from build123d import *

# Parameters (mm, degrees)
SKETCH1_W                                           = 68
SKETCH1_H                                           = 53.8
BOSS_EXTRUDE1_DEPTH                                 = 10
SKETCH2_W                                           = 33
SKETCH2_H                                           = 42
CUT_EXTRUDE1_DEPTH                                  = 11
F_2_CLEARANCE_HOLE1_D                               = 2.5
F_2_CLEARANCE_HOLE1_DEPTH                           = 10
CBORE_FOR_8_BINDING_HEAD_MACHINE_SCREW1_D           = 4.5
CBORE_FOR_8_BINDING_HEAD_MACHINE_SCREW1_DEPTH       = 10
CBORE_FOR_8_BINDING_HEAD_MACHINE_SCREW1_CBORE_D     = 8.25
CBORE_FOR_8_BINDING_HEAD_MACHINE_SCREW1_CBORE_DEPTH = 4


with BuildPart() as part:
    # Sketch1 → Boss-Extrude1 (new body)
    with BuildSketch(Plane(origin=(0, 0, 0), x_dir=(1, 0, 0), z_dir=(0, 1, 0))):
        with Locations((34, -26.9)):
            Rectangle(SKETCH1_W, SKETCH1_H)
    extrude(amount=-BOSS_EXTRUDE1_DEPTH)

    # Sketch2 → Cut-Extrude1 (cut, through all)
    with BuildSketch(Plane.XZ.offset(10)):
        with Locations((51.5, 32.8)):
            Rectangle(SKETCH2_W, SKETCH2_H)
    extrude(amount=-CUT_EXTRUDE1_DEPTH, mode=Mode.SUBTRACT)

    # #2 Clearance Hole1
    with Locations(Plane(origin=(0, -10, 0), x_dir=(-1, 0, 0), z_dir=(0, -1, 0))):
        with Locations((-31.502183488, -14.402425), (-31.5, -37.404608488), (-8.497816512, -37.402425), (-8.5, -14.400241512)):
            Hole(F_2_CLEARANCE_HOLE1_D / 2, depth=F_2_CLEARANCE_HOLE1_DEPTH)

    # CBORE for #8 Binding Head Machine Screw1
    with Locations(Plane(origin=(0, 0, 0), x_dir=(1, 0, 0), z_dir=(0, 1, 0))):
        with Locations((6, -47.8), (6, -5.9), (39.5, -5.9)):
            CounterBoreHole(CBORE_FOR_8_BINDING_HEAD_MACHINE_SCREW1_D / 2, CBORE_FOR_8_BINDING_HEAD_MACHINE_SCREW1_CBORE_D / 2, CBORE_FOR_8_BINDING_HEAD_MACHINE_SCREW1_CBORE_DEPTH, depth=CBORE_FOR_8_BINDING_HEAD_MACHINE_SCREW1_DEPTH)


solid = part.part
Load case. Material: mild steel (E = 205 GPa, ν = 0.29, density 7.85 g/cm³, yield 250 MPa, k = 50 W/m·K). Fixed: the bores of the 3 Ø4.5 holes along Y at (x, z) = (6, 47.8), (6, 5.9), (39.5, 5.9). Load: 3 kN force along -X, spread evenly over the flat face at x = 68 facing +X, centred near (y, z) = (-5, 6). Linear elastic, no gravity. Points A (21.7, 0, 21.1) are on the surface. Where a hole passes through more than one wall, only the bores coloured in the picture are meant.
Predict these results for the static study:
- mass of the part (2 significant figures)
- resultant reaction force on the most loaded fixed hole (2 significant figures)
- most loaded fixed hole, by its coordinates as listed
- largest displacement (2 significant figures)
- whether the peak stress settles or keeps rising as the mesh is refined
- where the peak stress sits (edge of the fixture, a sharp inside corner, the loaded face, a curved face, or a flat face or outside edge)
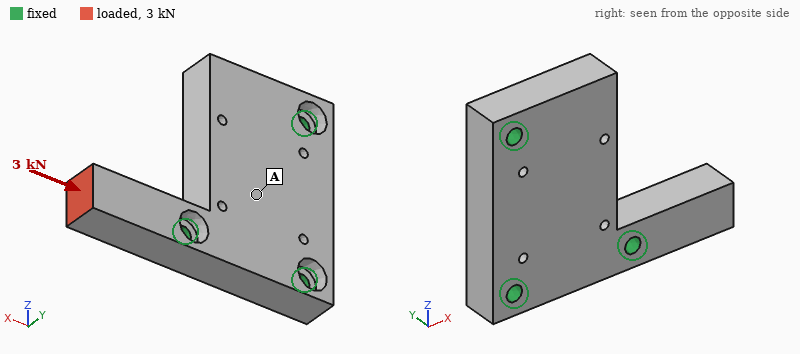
170 g
2.7 kN
(39.5, 5.9)
9.2 µm
keeps rising
edge of the fixture
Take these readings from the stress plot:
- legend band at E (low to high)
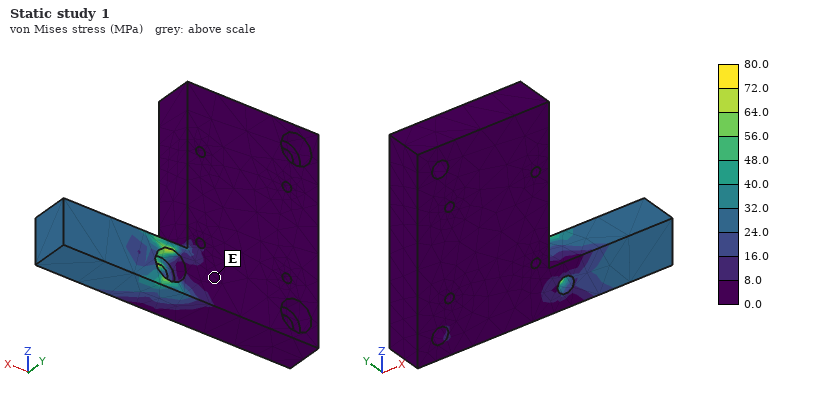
0.0 to 8.0 MPa
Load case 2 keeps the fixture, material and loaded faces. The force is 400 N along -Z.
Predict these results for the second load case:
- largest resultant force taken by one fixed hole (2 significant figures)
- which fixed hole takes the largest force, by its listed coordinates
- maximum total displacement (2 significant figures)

640 N
(39.5, 5.9)
18 µm
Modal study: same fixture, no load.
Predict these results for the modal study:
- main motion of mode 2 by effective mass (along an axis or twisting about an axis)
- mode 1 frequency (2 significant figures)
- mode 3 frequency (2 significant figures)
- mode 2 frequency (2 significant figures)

along Y
7400 Hz
8800 Hz
8200 Hz
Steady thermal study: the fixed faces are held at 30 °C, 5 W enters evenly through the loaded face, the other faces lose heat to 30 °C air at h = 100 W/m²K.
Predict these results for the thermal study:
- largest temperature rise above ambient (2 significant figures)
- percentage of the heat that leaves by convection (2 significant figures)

21 K
27 %
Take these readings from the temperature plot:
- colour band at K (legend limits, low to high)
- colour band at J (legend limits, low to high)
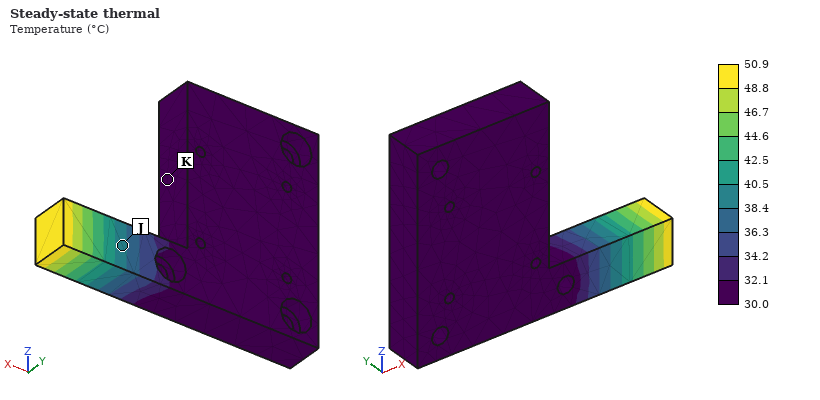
30.0 to 32.1 °C
38.4 to 40.5 °C
